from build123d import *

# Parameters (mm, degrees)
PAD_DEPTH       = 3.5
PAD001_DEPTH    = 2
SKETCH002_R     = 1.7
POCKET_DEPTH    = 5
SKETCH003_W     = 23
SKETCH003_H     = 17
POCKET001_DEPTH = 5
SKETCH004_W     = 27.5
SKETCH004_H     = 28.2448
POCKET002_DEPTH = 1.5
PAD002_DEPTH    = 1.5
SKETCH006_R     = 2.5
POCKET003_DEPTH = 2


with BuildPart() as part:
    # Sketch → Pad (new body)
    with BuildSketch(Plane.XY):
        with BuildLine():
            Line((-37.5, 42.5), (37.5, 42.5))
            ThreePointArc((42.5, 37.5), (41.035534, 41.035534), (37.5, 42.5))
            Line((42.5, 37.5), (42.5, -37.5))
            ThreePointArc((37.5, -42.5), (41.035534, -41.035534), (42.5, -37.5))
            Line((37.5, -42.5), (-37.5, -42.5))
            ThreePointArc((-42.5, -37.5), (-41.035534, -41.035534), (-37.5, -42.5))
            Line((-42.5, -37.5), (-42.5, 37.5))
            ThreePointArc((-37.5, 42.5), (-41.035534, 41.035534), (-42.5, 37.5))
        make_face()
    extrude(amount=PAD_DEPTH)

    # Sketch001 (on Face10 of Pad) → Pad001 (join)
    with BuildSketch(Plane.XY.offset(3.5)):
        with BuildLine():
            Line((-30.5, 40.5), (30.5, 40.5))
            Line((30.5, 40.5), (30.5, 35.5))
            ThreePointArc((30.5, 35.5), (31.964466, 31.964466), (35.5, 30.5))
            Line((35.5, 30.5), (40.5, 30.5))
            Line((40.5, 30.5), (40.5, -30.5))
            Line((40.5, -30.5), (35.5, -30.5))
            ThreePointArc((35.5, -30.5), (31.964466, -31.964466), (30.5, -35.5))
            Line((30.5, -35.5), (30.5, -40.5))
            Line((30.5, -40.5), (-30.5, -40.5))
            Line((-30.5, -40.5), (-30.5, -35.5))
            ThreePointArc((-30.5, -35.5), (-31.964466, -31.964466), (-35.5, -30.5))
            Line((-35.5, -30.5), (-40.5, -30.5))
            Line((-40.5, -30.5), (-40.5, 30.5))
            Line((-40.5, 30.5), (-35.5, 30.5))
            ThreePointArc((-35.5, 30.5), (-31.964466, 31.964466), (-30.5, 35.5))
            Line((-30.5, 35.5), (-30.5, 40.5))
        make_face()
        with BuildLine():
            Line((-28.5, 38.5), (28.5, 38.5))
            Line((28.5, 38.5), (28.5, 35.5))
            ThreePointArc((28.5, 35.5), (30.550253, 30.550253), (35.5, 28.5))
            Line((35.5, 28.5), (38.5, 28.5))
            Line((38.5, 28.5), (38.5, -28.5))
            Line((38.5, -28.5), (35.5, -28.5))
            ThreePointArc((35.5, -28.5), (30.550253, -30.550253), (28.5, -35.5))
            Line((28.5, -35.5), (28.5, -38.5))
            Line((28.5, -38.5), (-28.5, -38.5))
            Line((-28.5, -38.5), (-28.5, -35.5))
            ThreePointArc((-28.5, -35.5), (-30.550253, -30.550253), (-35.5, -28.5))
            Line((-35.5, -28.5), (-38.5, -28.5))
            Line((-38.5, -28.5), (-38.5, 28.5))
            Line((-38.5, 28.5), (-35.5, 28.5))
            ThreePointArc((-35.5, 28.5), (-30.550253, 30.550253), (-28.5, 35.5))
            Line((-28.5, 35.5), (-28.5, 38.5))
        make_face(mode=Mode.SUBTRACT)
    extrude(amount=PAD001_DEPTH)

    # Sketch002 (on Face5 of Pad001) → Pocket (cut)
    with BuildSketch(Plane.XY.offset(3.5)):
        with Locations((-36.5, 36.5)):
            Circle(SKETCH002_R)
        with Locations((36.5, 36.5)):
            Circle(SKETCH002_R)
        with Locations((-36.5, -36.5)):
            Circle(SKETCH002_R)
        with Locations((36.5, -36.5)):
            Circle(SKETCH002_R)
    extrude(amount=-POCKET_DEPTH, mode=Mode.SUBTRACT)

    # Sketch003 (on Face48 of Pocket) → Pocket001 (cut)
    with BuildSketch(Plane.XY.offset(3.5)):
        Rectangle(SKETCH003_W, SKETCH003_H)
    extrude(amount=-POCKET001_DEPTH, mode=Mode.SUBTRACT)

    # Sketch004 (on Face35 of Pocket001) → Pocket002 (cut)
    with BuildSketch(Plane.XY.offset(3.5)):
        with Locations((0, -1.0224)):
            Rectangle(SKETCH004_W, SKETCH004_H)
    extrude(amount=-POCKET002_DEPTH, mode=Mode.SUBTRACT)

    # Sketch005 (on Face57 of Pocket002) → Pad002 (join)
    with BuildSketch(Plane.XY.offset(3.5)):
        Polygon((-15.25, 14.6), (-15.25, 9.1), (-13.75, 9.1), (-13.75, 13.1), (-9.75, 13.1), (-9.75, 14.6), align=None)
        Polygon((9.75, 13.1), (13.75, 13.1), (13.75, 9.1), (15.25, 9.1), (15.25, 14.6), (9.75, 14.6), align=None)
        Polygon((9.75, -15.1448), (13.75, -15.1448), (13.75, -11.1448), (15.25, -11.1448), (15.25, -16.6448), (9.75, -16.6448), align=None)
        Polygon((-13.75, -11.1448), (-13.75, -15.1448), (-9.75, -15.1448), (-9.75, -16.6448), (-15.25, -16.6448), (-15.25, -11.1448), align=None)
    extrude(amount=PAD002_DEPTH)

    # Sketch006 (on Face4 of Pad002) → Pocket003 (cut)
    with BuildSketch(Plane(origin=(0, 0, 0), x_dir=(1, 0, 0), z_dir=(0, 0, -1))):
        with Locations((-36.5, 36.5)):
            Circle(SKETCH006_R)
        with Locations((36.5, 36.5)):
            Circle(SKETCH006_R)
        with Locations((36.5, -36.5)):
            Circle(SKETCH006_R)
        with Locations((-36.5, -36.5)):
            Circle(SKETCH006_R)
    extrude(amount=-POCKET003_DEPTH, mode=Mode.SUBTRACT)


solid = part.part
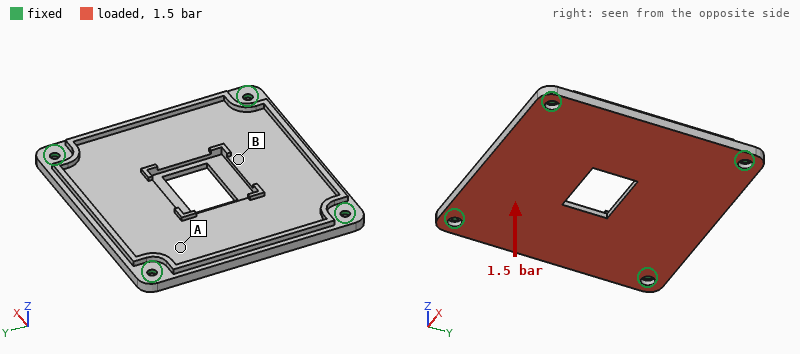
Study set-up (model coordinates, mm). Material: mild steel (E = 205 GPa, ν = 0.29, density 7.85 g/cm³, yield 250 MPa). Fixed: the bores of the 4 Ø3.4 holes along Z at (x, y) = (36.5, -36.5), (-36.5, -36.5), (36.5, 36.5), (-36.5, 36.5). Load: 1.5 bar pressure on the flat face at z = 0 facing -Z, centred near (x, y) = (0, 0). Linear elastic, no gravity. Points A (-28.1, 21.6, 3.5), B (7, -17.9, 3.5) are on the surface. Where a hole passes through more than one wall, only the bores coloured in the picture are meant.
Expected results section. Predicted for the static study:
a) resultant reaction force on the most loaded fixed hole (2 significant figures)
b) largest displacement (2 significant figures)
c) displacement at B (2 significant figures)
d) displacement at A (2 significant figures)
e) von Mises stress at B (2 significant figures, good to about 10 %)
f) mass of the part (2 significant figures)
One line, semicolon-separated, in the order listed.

520 N; 65 µm; 51 µm; 25 µm; 25 MPa; 190 g
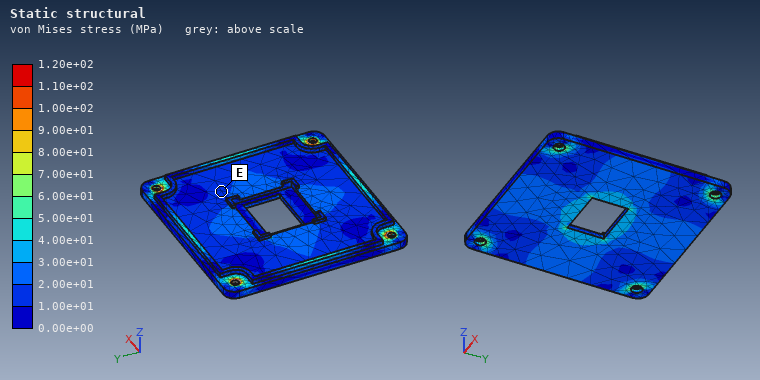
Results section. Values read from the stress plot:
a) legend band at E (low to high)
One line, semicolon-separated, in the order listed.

1.00e+01 to 2.00e+01 MPa
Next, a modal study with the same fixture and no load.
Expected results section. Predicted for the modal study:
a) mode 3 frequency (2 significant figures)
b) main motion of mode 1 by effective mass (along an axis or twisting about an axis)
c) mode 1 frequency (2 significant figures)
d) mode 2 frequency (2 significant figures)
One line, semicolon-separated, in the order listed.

3300 Hz; along Z; 1900 Hz; 3300 Hz
